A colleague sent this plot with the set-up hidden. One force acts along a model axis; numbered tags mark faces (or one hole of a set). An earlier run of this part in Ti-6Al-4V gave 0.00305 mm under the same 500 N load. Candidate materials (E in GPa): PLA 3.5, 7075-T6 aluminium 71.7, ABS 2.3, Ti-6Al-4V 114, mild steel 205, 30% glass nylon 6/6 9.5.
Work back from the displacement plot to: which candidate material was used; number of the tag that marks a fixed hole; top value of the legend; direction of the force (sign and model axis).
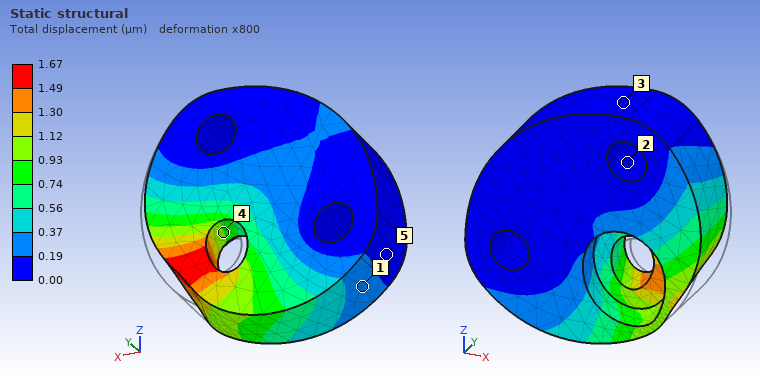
mild steel
2
1.67 µm
-X
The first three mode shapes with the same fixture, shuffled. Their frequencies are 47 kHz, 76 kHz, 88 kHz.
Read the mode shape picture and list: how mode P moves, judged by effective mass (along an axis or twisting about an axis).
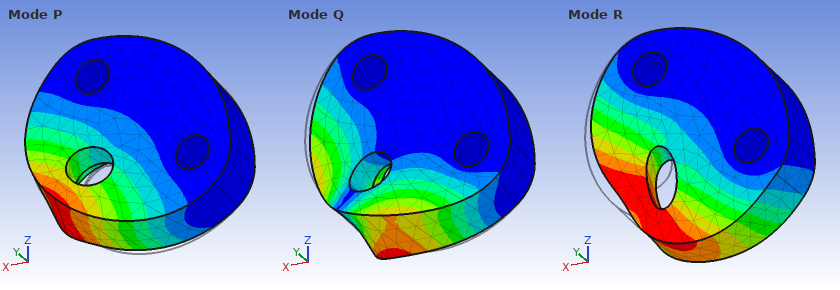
along Y
